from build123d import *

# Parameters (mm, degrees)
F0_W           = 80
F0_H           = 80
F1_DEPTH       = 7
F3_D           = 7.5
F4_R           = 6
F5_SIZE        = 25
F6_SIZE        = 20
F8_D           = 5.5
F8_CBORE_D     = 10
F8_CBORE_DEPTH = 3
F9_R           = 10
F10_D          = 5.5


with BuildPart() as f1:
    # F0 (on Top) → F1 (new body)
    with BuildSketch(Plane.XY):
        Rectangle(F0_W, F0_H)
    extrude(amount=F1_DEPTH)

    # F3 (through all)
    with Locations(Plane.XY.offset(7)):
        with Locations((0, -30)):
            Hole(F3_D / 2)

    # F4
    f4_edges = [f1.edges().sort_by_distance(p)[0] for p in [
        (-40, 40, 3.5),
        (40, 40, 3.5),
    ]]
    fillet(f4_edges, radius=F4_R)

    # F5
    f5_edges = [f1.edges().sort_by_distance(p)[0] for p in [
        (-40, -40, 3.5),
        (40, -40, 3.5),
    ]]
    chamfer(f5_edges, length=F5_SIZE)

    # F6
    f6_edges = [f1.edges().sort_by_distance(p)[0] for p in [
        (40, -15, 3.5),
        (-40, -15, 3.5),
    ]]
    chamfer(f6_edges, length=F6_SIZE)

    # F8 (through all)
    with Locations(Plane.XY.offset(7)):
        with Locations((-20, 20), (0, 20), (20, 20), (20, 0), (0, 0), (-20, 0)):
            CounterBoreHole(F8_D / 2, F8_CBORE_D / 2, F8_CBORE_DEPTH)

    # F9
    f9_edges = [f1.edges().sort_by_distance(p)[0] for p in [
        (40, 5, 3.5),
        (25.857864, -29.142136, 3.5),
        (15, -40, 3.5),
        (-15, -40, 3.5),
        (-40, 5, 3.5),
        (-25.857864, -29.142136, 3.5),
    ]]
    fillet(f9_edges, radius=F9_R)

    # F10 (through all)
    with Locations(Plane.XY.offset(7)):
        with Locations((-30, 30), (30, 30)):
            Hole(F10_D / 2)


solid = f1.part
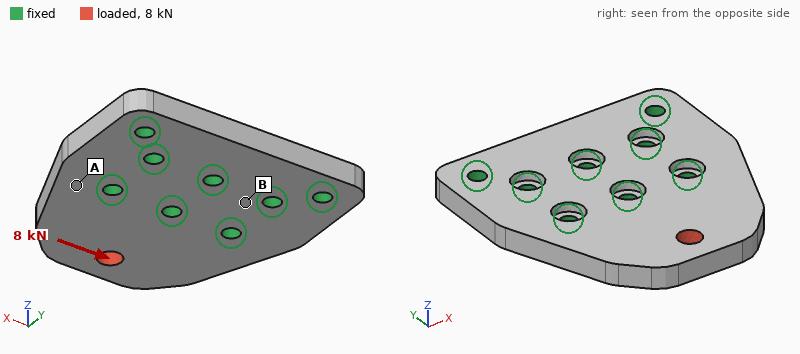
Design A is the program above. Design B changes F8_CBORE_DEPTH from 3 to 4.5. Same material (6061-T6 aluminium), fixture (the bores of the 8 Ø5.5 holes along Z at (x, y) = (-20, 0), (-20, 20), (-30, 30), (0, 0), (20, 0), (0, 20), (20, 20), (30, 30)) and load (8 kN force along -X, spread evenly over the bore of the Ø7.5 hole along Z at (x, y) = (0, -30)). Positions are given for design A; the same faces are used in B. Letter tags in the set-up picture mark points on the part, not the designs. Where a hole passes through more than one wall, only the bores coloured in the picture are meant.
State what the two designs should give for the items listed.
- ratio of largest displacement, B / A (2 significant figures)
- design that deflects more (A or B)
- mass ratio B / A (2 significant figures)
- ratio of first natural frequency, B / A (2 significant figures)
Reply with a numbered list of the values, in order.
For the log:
1. 1.1
2. B
3. 0.99
4. 0.94
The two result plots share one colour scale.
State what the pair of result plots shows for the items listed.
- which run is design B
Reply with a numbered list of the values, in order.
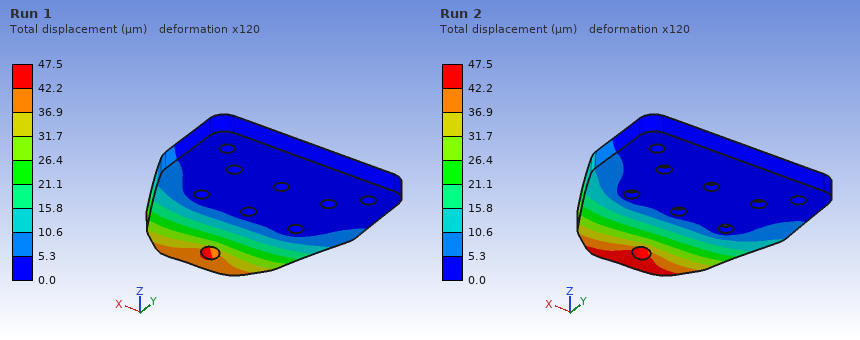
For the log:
1. Run 2
